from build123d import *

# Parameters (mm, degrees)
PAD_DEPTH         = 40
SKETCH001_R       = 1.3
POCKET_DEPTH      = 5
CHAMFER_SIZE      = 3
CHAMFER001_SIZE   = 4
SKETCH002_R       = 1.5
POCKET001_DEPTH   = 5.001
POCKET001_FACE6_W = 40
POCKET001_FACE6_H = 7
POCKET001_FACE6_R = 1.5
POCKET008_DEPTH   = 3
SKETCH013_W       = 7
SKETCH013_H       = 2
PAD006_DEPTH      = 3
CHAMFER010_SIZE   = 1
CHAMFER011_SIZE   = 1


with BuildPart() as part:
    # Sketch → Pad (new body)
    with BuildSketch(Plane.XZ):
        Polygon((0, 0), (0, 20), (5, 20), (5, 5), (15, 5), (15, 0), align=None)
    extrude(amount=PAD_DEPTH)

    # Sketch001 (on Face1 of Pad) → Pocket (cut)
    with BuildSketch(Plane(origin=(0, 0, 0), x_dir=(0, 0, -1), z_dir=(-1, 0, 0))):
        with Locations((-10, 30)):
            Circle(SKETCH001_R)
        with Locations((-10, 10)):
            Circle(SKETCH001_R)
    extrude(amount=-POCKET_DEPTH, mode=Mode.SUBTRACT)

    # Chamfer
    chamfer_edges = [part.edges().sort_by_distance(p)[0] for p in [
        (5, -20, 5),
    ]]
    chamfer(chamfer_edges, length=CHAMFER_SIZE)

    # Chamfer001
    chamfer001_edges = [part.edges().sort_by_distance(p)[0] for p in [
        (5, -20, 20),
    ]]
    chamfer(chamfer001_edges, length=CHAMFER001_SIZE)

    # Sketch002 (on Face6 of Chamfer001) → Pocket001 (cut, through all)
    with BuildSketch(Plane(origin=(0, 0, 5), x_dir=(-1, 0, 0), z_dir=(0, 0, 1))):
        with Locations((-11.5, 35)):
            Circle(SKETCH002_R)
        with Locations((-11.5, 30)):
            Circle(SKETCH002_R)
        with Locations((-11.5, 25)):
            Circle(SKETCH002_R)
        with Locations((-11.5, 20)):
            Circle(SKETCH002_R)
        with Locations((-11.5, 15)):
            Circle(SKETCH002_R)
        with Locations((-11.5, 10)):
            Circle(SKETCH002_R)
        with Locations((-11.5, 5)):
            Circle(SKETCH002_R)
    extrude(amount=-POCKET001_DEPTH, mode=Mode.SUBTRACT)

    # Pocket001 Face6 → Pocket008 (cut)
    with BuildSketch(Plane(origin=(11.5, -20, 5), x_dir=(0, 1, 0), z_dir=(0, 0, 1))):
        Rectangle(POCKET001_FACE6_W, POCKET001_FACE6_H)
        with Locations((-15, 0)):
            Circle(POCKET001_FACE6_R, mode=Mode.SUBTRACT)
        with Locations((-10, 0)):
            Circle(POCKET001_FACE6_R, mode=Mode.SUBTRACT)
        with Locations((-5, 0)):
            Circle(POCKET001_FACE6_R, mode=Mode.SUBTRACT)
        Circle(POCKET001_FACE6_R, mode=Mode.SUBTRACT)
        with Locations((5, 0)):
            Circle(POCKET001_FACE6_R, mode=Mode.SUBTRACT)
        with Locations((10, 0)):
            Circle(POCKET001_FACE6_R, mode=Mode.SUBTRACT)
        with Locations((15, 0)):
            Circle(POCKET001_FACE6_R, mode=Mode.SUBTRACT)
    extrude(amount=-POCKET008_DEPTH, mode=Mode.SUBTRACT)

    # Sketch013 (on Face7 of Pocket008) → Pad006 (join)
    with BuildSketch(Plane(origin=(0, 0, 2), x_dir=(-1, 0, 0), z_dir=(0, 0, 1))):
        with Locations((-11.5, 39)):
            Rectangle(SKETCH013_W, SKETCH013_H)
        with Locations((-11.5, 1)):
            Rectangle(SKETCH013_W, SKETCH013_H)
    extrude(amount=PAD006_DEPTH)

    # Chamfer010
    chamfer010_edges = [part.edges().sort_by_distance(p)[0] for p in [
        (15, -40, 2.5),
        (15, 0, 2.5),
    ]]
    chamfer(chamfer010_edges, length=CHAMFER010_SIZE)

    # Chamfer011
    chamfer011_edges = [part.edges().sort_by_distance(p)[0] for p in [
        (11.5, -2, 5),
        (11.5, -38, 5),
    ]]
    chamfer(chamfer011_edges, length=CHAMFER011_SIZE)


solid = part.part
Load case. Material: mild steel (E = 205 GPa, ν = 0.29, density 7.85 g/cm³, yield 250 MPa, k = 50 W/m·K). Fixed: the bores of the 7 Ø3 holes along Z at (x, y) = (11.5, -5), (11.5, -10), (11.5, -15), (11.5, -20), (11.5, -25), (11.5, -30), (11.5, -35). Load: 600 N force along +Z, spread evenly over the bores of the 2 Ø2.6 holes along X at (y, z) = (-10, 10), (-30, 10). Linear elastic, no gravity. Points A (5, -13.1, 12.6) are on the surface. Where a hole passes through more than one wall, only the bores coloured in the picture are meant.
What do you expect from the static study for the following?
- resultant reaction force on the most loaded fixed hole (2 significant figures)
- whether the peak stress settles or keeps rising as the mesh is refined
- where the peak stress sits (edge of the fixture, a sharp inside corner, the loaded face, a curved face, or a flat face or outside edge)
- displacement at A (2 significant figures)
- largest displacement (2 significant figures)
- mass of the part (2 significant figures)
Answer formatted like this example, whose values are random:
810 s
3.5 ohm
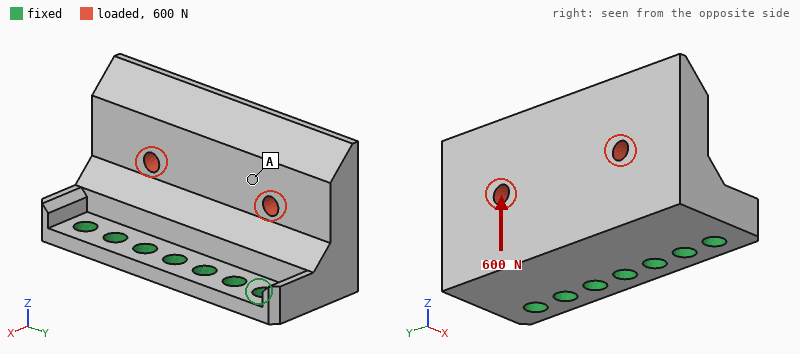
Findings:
120 N
keeps rising
edge of the fixture
21 µm
36 µm
39 g
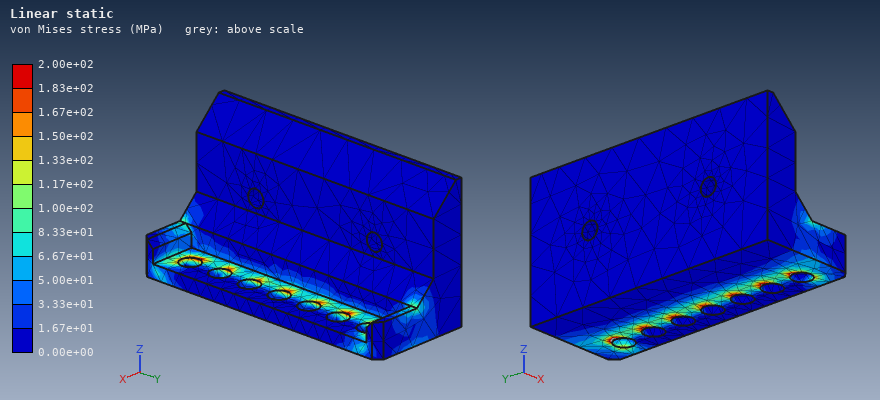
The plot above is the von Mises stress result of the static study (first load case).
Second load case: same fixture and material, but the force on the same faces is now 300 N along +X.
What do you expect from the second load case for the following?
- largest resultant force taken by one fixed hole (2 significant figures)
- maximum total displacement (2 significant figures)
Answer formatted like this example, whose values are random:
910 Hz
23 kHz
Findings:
90 N
26 µm
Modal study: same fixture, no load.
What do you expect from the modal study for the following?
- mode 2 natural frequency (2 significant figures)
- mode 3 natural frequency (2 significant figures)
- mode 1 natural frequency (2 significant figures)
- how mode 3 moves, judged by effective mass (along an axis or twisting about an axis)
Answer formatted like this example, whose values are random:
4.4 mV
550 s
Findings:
10 kHz
19 kHz
3700 Hz
along Y
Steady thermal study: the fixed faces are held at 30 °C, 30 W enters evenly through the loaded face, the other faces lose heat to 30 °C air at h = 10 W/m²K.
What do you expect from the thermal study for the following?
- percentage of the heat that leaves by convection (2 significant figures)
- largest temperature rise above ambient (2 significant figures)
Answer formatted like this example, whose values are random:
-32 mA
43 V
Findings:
3.2 %
63 K
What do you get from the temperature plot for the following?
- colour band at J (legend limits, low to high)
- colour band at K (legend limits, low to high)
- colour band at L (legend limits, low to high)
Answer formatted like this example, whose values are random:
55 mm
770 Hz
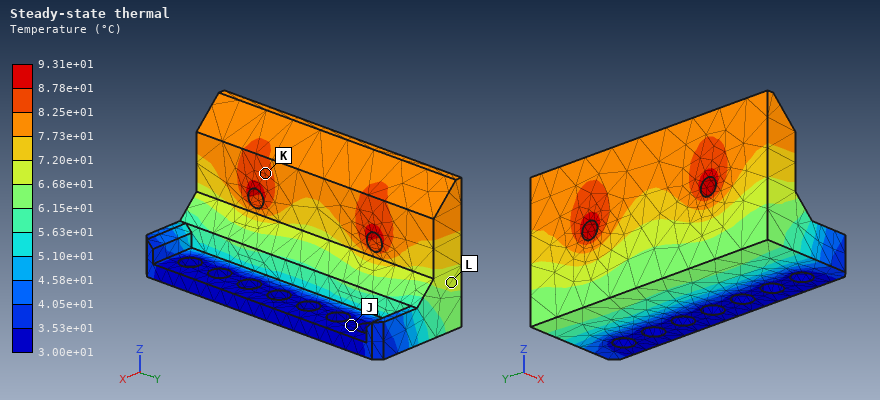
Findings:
3.00e+01 to 3.53e+01 °C
8.25e+01 to 8.78e+01 °C
6.68e+01 to 7.20e+01 °C
